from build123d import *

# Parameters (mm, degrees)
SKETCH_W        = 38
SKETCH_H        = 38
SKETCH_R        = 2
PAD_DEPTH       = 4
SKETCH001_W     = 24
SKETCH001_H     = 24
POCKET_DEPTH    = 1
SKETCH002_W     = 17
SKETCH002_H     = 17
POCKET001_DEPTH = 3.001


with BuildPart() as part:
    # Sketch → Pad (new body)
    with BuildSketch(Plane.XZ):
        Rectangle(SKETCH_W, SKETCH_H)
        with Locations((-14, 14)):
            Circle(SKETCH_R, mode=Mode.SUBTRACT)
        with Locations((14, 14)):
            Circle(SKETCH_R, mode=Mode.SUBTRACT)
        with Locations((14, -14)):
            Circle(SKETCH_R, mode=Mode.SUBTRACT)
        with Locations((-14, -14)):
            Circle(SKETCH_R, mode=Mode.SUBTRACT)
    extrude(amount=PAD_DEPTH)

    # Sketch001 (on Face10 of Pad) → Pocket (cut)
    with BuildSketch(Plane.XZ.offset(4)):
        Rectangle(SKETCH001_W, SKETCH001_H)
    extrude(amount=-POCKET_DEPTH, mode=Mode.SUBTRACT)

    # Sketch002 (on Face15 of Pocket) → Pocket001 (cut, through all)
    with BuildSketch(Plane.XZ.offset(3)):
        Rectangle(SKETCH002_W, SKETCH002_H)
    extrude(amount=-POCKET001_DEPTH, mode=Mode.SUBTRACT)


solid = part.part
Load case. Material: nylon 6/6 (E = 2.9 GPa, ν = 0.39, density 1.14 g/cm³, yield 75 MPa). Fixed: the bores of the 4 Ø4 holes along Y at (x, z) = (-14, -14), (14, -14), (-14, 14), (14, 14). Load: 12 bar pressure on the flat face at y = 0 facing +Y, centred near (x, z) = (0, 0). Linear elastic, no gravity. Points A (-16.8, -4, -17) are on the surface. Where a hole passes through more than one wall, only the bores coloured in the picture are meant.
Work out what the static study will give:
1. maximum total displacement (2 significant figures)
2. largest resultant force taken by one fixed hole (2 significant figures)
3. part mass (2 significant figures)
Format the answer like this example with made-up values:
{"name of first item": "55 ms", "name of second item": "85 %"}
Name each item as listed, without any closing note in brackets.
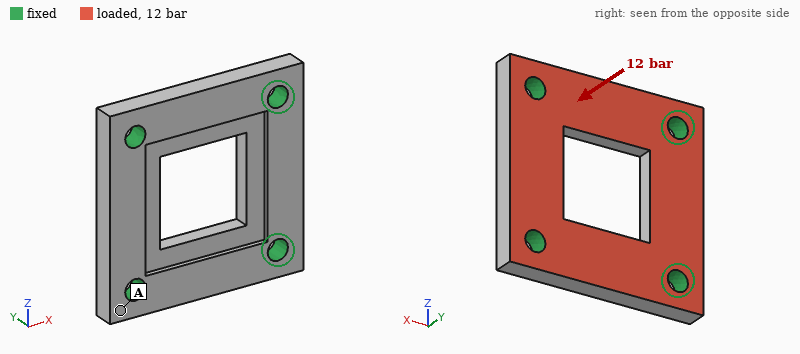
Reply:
{"maximum total displacement": "0.18 mm", "largest resultant force taken by one fixed hole": "330 N", "part mass": "4.7 g"}
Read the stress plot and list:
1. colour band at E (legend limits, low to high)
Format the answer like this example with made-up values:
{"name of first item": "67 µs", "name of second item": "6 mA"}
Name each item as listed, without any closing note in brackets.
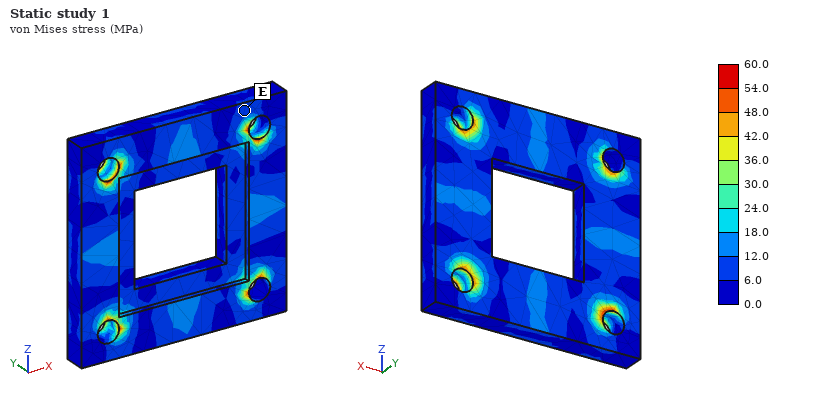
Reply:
{"colour band at E": "6.0 to 12.0 MPa"}
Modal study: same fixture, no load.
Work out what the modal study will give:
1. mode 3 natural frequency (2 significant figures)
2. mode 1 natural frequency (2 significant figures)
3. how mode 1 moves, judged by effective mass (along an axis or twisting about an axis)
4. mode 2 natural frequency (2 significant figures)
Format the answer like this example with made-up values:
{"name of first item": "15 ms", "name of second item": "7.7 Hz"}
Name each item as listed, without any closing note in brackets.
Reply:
{"mode 3 natural frequency": "8500 Hz", "mode 1 natural frequency": "8200 Hz", "how mode 1 moves, judged by effective mass": "along Y", "mode 2 natural frequency": "8500 Hz"}
